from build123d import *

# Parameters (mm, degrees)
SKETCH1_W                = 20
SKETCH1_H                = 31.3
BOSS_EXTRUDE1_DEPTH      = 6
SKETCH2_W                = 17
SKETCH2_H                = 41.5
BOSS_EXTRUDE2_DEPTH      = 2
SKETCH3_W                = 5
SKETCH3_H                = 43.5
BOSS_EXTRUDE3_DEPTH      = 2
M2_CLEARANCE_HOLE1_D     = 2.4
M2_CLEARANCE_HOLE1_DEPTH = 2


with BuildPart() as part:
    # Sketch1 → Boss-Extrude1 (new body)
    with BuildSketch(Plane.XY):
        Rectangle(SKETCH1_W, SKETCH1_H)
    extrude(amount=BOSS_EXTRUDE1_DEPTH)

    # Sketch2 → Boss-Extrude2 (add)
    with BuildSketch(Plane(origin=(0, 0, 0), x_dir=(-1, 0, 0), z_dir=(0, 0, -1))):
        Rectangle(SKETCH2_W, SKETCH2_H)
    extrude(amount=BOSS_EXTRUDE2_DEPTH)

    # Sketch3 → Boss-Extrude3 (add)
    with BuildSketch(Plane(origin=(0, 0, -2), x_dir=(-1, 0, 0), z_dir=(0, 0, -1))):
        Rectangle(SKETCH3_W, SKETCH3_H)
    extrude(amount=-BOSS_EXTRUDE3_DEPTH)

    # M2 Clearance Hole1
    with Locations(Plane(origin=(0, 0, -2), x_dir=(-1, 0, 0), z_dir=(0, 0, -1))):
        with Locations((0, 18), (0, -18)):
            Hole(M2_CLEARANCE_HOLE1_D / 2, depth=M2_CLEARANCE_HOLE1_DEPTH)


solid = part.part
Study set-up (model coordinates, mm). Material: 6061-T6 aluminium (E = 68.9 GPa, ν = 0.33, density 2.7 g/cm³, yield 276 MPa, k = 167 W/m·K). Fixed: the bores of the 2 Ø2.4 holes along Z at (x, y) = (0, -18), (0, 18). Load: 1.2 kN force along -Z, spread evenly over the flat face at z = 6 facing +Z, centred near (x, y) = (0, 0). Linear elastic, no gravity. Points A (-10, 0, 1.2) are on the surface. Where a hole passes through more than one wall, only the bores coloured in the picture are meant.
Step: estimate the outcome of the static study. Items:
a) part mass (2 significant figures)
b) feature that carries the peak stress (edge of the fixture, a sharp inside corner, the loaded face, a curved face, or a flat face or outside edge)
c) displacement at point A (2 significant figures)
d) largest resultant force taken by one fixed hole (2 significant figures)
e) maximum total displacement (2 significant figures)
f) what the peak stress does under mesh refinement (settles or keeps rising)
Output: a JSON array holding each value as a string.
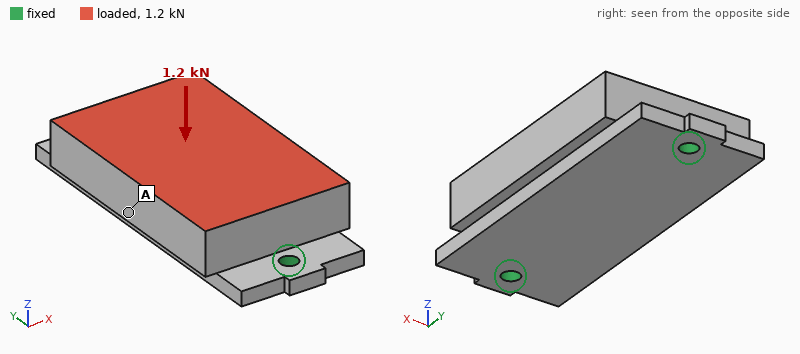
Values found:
["14 g", "edge of the fixture", "17 µm", "770 N", "17 µm", "keeps rising"]
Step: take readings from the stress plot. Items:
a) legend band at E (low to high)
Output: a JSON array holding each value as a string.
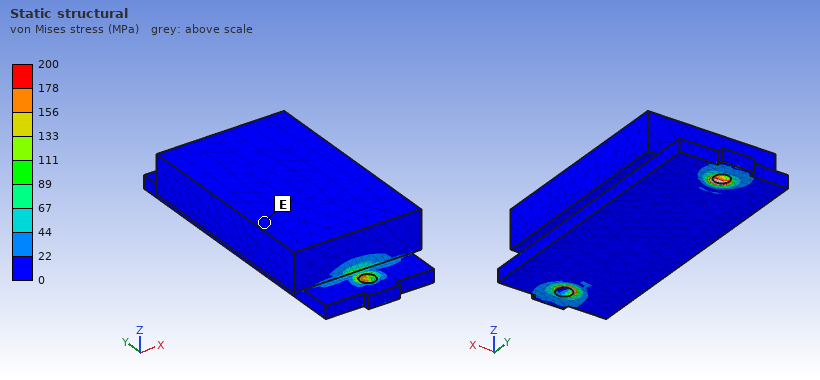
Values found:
["0 to 22 MPa"]
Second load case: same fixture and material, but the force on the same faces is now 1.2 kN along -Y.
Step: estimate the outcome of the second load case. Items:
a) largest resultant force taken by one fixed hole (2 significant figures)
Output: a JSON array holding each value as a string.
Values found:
["650 N"]
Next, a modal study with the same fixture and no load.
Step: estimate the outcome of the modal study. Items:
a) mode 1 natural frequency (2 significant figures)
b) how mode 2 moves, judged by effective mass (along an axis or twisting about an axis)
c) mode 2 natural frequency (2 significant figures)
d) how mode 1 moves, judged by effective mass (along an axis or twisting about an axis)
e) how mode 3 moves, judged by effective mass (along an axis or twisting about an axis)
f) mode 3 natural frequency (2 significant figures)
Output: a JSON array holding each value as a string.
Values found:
["5400 Hz", "along Z", "13 kHz", "along X", "along X", "22 kHz"]
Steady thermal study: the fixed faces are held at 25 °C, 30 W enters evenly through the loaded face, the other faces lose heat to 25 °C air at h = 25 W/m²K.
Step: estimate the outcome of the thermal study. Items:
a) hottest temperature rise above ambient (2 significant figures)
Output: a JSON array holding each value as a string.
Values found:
["21 K"]
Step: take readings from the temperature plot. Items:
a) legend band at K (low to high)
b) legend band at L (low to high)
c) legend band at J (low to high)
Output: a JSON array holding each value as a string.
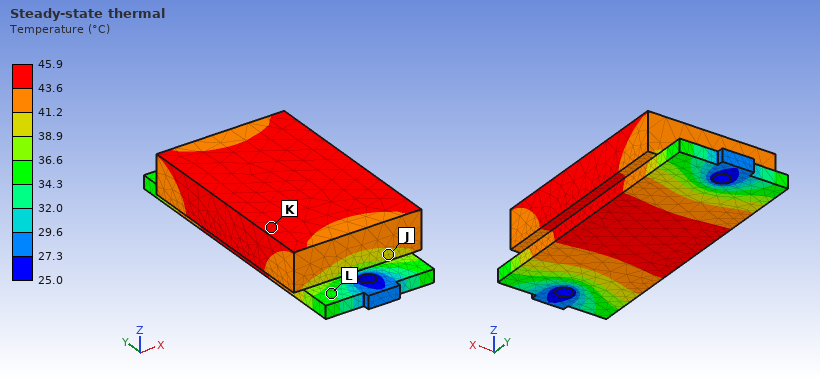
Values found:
["43.6 to 45.9 °C", "34.3 to 36.6 °C", "38.9 to 41.2 °C"]
